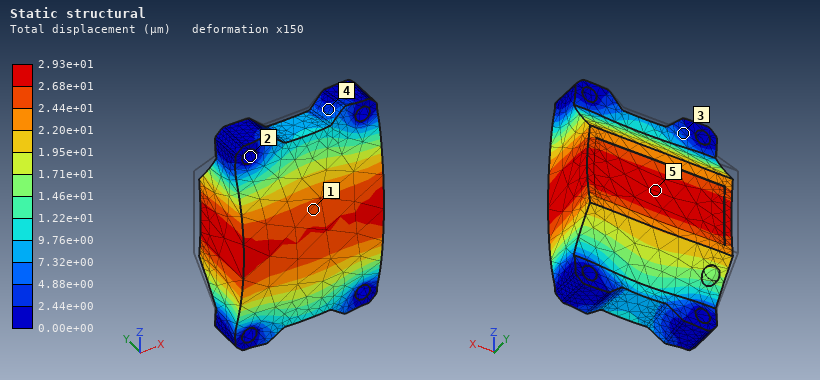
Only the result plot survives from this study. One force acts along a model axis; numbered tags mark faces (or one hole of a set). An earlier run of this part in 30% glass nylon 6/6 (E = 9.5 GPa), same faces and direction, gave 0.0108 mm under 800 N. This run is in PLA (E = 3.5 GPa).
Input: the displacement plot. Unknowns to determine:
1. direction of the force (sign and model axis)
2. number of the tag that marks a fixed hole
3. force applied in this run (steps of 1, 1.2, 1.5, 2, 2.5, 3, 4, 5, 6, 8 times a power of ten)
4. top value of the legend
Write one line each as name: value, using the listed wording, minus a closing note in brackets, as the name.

direction of the force: -Y
number of the tag that marks a fixed hole: 2
force applied in this run: 800 N
top value of the legend: 2.93e+01 µm
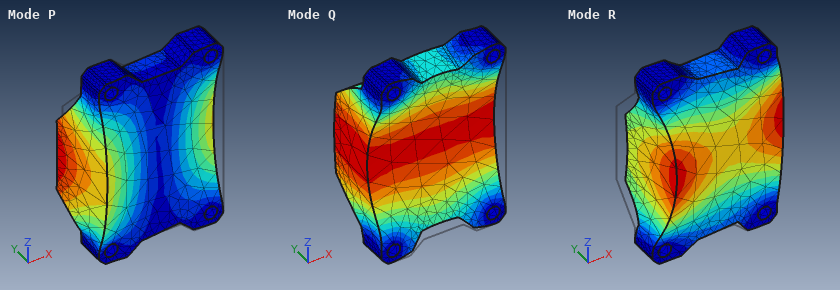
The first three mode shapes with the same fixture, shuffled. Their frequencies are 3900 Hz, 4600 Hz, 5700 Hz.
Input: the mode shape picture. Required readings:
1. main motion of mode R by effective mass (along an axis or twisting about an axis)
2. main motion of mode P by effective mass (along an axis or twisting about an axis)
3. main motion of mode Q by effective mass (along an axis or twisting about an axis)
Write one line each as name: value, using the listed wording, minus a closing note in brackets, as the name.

main motion of mode R by effective mass: along X
main motion of mode P by effective mass: along X
main motion of mode Q by effective mass: along Y
